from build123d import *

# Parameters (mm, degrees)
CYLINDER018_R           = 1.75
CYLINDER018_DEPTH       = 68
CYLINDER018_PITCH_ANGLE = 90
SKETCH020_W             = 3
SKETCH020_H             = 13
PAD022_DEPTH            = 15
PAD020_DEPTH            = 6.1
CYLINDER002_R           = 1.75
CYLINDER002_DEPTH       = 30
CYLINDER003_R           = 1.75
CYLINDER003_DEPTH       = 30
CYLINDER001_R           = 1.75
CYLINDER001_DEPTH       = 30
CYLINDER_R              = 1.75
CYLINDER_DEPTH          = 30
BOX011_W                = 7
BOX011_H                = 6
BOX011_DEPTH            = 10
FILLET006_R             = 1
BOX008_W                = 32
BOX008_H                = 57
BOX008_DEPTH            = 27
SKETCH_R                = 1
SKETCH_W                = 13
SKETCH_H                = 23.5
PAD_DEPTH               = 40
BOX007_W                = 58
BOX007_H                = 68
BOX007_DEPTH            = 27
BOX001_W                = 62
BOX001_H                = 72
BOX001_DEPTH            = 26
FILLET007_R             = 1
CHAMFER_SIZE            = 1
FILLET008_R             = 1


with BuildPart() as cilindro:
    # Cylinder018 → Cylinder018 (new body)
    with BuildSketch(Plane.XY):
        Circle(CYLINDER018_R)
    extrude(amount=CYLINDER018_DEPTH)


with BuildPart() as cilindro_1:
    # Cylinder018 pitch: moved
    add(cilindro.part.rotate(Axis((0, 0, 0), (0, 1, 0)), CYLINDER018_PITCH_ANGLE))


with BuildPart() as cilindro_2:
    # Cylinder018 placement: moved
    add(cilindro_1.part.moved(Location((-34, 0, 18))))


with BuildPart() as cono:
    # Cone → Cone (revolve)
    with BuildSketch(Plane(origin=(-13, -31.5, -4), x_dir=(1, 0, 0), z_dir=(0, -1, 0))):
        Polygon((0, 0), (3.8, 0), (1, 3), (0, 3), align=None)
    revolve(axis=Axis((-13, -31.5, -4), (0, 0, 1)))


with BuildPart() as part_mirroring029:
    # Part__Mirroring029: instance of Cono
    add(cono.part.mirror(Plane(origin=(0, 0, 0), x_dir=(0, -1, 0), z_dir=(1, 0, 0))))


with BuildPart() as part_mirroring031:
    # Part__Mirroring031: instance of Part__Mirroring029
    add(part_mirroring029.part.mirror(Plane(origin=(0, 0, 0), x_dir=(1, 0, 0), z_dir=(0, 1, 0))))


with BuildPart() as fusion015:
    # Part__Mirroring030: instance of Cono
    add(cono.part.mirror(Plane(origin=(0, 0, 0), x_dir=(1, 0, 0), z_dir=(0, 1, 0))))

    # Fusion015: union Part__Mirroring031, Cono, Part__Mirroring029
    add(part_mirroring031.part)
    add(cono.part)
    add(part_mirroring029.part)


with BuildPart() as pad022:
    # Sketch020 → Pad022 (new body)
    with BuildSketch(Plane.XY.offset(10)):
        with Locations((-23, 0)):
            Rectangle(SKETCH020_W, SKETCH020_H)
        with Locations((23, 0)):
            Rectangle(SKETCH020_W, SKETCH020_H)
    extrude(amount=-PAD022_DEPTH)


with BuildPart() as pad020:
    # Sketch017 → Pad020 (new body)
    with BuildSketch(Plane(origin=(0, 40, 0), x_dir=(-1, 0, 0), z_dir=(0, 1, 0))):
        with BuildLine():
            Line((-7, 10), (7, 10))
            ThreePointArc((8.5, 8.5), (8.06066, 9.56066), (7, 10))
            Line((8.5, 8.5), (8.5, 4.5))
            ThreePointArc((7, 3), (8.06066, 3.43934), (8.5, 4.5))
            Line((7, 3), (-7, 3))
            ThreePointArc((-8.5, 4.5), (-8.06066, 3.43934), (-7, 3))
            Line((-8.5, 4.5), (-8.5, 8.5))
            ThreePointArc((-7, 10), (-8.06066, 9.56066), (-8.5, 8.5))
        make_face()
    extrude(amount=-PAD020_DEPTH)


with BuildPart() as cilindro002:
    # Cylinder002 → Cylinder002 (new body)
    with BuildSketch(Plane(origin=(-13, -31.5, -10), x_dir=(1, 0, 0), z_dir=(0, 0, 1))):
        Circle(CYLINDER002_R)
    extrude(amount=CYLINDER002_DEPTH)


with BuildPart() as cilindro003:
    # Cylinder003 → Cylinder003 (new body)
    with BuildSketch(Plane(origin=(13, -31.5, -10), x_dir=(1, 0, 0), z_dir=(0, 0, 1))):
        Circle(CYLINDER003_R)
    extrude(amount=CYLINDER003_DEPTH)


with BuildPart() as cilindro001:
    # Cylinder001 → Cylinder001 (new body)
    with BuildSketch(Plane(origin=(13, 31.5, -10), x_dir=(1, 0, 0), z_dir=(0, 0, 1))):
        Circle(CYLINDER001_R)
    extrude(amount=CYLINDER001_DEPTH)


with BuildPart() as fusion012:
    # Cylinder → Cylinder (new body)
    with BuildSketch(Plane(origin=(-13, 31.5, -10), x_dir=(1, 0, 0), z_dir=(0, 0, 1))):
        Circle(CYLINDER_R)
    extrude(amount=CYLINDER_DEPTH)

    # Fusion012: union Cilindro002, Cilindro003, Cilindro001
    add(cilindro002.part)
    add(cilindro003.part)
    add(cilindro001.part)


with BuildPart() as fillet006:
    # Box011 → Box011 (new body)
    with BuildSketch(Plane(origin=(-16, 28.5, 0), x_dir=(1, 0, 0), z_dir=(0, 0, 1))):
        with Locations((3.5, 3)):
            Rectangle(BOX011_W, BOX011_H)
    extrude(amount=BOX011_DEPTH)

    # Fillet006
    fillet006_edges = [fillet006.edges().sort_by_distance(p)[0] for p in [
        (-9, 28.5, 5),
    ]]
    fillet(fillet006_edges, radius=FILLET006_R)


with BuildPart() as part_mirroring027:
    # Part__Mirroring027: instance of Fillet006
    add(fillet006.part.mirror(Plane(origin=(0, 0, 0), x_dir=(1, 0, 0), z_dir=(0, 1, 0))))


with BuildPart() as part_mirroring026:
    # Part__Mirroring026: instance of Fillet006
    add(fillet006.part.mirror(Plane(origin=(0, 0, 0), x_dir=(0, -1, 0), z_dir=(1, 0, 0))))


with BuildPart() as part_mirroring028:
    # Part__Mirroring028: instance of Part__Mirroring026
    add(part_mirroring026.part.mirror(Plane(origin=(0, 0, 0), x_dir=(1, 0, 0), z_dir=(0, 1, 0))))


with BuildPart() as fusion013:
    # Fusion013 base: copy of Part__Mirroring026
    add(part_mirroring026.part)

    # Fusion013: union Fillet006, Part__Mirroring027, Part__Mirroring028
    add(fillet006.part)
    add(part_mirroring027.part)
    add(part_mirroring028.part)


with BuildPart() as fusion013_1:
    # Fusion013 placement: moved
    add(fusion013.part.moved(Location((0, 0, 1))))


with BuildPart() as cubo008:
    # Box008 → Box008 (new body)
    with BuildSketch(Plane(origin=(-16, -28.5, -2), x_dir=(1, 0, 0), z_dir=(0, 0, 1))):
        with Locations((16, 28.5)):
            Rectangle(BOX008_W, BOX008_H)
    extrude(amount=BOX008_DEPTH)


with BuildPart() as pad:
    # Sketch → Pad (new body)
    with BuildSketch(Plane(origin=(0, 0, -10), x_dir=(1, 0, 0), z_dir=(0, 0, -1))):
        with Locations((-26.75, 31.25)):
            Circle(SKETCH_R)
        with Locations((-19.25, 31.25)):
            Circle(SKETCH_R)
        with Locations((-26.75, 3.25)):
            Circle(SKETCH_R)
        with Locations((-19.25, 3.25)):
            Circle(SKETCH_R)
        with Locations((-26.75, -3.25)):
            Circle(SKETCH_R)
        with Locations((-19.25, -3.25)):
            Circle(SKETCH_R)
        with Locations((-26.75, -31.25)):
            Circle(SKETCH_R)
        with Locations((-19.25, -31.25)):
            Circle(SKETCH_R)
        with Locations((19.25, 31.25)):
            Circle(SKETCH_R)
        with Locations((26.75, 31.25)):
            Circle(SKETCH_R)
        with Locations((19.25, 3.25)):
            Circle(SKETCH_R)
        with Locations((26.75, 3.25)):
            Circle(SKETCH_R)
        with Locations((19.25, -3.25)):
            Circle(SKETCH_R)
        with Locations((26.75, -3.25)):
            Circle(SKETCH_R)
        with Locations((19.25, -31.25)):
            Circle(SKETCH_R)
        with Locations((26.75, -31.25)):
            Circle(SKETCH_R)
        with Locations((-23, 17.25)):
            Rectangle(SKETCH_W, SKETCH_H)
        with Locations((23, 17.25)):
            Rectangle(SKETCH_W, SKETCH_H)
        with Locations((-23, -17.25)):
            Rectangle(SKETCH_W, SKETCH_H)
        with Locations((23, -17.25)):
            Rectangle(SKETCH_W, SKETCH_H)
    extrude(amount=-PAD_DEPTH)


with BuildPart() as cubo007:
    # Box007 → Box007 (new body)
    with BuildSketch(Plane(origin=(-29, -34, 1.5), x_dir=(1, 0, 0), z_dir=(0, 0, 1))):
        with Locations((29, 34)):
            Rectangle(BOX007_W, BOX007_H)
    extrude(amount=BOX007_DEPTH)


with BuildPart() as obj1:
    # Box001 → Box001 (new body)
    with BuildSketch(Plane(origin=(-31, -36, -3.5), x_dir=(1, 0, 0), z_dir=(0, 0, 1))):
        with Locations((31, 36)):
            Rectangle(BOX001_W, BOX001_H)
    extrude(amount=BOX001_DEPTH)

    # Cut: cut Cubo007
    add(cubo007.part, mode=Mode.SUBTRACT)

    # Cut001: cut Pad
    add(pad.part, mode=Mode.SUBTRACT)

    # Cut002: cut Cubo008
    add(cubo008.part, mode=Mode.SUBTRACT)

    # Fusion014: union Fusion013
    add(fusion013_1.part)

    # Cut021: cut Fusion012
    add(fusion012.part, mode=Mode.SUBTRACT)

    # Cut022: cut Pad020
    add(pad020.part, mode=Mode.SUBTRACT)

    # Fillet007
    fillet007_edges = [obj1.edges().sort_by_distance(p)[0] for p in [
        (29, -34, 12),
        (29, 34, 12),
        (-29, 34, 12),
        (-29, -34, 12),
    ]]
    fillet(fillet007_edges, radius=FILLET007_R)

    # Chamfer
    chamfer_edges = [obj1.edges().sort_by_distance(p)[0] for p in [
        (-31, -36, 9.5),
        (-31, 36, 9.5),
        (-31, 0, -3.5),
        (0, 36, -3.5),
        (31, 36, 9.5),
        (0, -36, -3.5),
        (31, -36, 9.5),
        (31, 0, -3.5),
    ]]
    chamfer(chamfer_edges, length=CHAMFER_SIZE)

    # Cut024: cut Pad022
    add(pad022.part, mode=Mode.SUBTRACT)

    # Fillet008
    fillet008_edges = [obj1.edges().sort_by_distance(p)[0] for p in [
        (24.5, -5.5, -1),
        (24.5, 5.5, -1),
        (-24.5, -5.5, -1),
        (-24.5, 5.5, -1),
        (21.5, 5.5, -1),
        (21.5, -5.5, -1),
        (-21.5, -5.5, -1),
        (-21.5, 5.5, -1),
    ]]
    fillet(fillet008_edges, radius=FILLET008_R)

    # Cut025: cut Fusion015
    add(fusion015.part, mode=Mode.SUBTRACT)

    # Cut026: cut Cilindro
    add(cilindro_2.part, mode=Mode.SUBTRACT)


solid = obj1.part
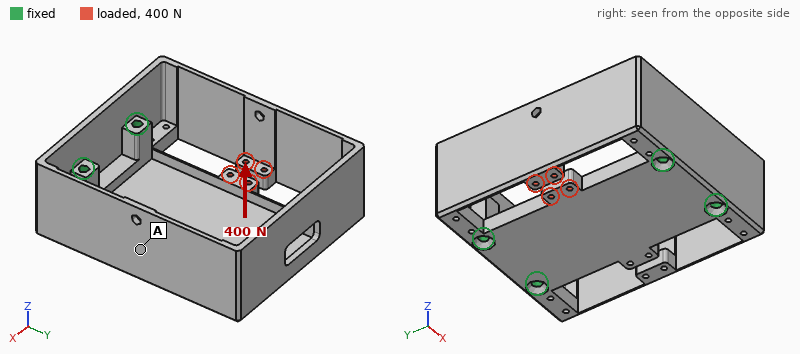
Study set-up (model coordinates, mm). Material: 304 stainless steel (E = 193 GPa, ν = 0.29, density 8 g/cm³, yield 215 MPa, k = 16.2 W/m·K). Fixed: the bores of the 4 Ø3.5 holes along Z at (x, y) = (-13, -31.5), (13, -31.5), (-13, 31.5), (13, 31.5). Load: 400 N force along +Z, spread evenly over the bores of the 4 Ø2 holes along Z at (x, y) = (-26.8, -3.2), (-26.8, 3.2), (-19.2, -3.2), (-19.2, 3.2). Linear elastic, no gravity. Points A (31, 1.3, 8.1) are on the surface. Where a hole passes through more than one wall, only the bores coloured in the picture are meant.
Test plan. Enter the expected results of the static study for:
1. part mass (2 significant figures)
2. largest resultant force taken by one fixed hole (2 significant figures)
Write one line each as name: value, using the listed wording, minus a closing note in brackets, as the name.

part mass: 160 g
largest resultant force taken by one fixed hole: 250 N
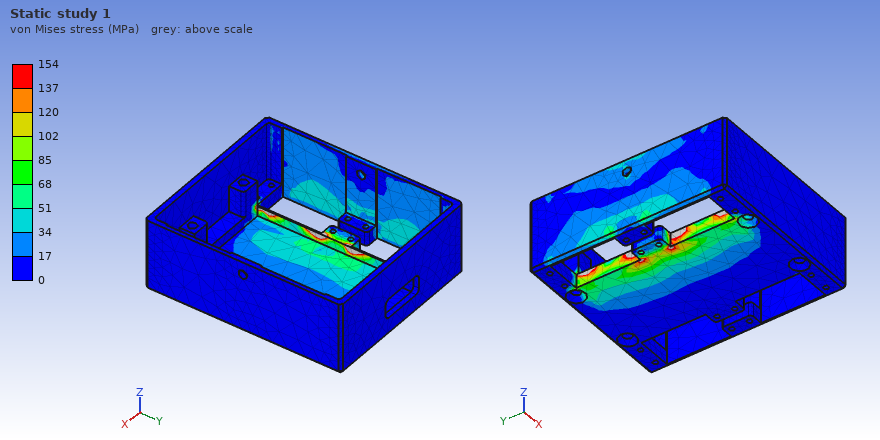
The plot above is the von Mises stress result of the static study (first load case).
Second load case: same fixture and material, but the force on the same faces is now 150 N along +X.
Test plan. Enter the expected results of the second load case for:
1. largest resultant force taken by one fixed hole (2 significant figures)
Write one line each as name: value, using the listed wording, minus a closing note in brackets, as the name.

largest resultant force taken by one fixed hole: 59 N
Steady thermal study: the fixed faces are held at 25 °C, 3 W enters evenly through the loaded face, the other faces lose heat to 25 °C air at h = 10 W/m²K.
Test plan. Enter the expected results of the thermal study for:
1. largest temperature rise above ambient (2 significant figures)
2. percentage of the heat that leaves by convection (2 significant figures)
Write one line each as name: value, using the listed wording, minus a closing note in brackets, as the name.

largest temperature rise above ambient: 48 K
percentage of the heat that leaves by convection: 46 %
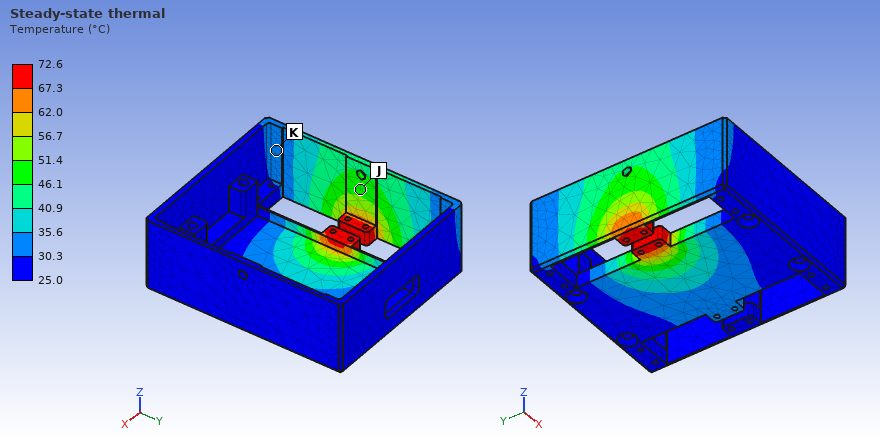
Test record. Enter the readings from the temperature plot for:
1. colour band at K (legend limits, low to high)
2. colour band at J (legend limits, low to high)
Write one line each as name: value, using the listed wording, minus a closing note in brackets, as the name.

colour band at K: 30.3 to 35.6 °C
colour band at J: 46.1 to 51.4 °C
